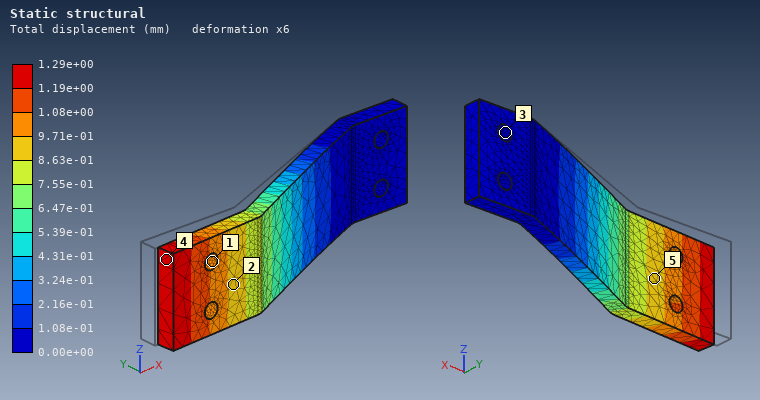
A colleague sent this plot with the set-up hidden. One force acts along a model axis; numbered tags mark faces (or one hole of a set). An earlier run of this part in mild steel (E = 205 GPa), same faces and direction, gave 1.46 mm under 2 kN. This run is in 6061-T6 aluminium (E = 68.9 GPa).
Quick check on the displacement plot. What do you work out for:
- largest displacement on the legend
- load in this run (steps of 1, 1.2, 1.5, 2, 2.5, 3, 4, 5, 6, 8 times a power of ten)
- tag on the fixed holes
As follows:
1.29e+00 mm
600 N
3
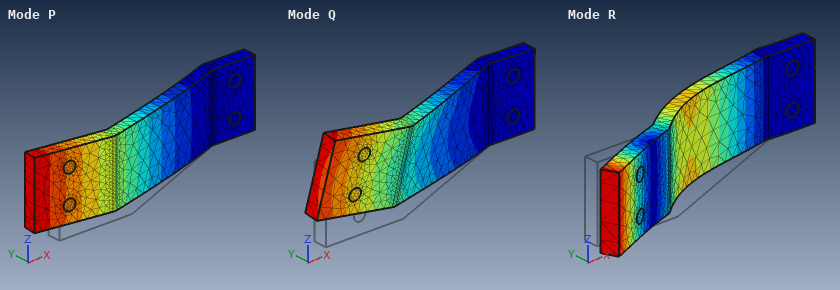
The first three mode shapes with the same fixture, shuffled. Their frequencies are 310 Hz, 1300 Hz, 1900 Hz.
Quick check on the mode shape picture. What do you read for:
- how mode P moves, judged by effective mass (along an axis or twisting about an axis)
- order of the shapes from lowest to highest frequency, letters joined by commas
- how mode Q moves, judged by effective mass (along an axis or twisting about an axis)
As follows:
along Y
P, Q, R
along Z
